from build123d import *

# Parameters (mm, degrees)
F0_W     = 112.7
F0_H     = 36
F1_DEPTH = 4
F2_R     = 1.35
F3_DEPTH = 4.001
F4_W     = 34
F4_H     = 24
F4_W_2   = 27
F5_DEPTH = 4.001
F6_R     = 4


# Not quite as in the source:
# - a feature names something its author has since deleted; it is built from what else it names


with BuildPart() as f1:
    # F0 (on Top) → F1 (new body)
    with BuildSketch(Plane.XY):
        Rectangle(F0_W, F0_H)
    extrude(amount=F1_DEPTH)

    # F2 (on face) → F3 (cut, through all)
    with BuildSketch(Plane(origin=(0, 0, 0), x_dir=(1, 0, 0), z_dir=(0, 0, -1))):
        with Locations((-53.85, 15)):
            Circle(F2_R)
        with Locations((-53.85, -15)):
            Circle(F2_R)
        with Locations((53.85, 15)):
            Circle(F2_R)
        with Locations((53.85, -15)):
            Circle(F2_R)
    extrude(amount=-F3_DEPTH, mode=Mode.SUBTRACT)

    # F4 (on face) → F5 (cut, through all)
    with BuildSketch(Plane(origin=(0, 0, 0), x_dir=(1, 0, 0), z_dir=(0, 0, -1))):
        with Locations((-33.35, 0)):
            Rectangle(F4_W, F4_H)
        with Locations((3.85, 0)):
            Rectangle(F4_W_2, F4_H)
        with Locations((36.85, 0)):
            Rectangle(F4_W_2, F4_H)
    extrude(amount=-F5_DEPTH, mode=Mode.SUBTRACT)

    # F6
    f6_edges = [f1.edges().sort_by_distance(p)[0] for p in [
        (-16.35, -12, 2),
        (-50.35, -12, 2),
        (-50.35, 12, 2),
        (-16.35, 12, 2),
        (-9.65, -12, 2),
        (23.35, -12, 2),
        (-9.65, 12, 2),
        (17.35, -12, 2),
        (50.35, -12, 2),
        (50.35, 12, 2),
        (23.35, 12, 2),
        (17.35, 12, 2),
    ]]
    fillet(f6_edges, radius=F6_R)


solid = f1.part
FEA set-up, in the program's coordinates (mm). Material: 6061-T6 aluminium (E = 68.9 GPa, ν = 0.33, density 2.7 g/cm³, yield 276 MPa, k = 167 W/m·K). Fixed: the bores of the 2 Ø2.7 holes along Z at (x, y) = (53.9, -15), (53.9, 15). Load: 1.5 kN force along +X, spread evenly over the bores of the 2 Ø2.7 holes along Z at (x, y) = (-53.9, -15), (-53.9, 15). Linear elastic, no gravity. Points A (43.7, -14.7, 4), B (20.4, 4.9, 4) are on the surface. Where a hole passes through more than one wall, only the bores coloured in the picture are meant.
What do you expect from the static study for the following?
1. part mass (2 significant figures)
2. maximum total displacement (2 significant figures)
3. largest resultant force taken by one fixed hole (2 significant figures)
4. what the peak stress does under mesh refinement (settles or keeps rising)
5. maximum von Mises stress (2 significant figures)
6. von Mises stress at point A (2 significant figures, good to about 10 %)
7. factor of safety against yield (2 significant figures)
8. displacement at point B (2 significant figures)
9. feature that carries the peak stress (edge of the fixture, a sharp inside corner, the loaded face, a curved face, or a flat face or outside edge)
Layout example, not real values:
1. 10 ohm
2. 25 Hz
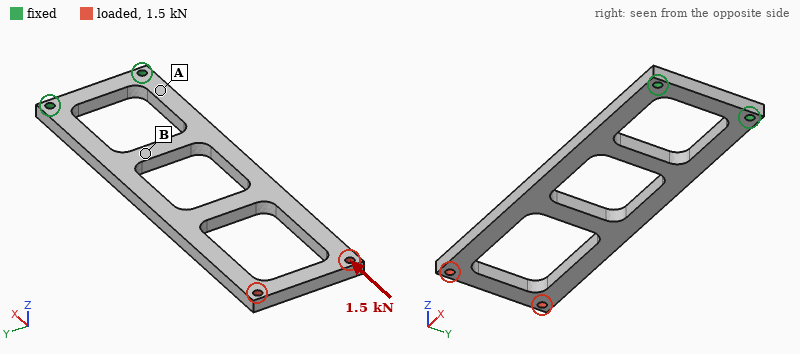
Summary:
1. 21 g
2. 50 µm
3. 750 N
4. settles
5. 87 MPa
6. 31 MPa
7. 3.2
8. 14 µm
9. the loaded face
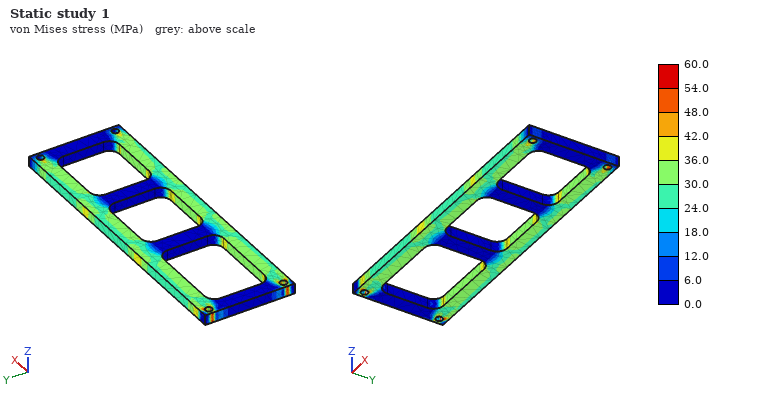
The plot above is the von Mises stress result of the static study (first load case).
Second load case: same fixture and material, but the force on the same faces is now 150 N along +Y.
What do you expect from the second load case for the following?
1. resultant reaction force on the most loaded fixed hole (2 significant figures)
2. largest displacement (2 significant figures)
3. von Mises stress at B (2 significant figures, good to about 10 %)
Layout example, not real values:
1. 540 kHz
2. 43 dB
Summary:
1. 490 N
2. 0.30 mm
3. 18 MPa
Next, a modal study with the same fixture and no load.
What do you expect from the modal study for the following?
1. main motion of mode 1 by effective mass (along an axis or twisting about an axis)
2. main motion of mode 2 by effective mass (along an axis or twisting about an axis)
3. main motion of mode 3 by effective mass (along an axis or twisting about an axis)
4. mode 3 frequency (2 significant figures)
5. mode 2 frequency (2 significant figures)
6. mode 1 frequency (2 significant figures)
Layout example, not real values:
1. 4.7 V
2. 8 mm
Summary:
1. along Z
2. twisting about X
3. along Y
4. 1400 Hz
5. 1100 Hz
6. 230 Hz
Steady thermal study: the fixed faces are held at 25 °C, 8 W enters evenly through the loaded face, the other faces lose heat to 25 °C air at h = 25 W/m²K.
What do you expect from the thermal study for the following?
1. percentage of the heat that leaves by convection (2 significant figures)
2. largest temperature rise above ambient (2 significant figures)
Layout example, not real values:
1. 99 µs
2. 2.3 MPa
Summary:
1. 53 %
2. 63 K
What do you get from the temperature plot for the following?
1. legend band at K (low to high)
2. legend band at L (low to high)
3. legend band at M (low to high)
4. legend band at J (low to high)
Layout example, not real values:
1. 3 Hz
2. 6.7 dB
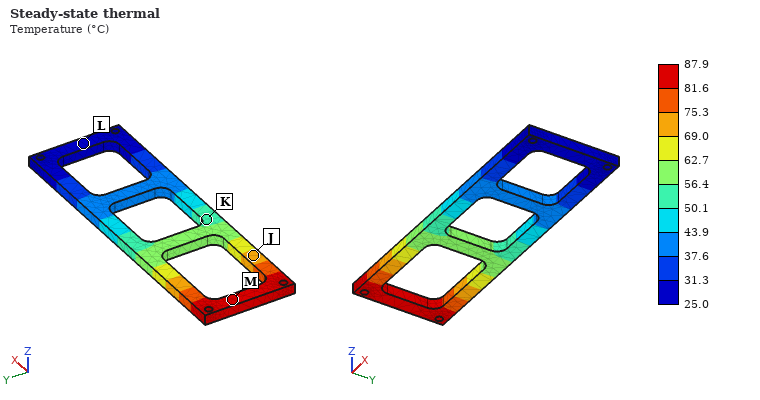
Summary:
1. 50.1 to 56.4 °C
2. 25.0 to 31.3 °C
3. 81.6 to 87.9 °C
4. 69.0 to 75.3 °C
